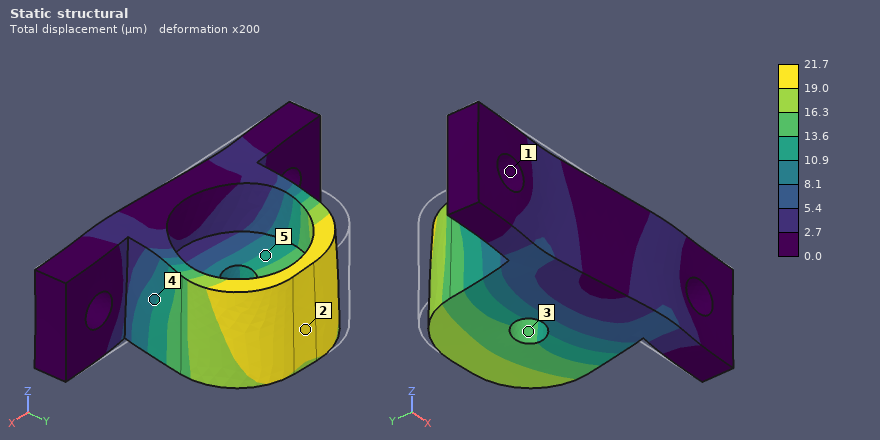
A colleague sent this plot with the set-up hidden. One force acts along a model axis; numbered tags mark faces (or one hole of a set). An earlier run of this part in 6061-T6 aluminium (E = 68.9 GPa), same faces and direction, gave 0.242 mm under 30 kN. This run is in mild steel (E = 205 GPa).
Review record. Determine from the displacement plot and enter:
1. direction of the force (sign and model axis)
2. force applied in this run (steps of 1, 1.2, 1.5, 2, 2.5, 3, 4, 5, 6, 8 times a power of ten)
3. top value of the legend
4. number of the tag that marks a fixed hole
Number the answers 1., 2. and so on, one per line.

1. +X
2. 8 kN
3. 21.7 µm
4. 1
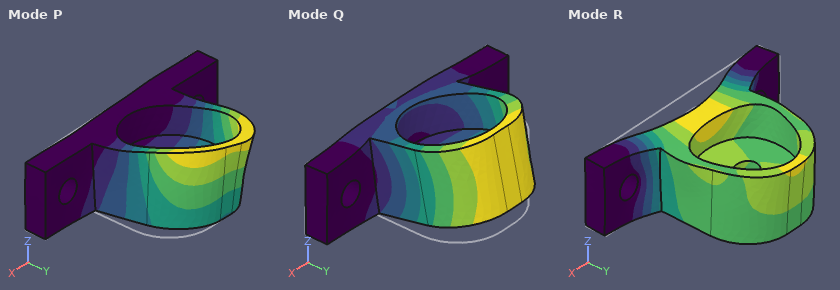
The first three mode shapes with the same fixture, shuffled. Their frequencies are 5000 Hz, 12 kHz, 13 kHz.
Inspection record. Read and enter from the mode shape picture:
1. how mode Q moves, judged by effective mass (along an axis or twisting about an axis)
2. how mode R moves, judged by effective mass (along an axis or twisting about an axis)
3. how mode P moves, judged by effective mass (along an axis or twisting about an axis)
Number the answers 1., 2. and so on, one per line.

1. along Z
2. along Y
3. along X
